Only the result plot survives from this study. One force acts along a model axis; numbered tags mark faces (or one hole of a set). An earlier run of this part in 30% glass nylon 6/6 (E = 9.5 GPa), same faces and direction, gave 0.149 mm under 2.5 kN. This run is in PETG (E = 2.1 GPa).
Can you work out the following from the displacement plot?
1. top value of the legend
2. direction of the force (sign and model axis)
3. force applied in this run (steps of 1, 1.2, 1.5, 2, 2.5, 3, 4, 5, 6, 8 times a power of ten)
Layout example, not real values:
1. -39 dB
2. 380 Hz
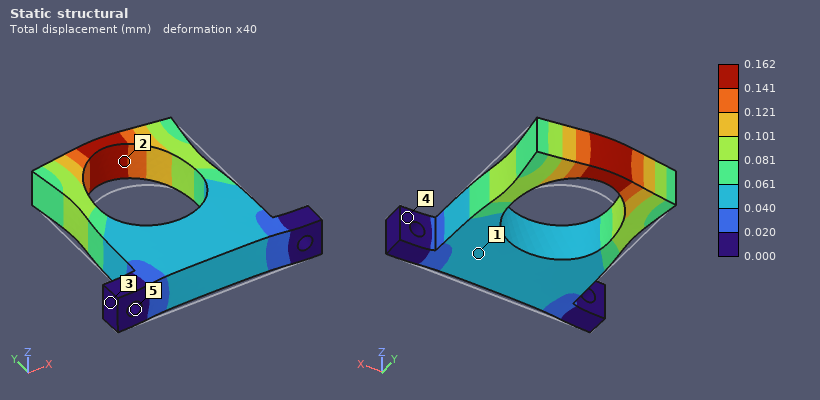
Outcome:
1. 0.162 mm
2. +Y
3. 600 N
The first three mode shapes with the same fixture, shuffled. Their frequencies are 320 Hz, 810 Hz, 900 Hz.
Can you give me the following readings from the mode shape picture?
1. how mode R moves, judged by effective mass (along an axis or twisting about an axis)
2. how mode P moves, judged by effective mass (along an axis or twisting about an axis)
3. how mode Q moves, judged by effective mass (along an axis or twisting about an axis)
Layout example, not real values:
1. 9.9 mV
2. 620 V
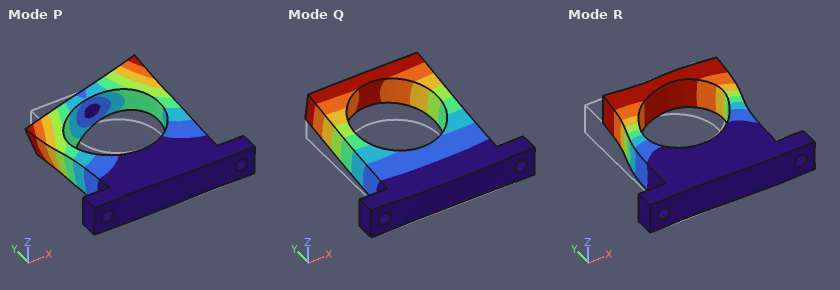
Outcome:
1. along X
2. twisting about Y
3. along Z
